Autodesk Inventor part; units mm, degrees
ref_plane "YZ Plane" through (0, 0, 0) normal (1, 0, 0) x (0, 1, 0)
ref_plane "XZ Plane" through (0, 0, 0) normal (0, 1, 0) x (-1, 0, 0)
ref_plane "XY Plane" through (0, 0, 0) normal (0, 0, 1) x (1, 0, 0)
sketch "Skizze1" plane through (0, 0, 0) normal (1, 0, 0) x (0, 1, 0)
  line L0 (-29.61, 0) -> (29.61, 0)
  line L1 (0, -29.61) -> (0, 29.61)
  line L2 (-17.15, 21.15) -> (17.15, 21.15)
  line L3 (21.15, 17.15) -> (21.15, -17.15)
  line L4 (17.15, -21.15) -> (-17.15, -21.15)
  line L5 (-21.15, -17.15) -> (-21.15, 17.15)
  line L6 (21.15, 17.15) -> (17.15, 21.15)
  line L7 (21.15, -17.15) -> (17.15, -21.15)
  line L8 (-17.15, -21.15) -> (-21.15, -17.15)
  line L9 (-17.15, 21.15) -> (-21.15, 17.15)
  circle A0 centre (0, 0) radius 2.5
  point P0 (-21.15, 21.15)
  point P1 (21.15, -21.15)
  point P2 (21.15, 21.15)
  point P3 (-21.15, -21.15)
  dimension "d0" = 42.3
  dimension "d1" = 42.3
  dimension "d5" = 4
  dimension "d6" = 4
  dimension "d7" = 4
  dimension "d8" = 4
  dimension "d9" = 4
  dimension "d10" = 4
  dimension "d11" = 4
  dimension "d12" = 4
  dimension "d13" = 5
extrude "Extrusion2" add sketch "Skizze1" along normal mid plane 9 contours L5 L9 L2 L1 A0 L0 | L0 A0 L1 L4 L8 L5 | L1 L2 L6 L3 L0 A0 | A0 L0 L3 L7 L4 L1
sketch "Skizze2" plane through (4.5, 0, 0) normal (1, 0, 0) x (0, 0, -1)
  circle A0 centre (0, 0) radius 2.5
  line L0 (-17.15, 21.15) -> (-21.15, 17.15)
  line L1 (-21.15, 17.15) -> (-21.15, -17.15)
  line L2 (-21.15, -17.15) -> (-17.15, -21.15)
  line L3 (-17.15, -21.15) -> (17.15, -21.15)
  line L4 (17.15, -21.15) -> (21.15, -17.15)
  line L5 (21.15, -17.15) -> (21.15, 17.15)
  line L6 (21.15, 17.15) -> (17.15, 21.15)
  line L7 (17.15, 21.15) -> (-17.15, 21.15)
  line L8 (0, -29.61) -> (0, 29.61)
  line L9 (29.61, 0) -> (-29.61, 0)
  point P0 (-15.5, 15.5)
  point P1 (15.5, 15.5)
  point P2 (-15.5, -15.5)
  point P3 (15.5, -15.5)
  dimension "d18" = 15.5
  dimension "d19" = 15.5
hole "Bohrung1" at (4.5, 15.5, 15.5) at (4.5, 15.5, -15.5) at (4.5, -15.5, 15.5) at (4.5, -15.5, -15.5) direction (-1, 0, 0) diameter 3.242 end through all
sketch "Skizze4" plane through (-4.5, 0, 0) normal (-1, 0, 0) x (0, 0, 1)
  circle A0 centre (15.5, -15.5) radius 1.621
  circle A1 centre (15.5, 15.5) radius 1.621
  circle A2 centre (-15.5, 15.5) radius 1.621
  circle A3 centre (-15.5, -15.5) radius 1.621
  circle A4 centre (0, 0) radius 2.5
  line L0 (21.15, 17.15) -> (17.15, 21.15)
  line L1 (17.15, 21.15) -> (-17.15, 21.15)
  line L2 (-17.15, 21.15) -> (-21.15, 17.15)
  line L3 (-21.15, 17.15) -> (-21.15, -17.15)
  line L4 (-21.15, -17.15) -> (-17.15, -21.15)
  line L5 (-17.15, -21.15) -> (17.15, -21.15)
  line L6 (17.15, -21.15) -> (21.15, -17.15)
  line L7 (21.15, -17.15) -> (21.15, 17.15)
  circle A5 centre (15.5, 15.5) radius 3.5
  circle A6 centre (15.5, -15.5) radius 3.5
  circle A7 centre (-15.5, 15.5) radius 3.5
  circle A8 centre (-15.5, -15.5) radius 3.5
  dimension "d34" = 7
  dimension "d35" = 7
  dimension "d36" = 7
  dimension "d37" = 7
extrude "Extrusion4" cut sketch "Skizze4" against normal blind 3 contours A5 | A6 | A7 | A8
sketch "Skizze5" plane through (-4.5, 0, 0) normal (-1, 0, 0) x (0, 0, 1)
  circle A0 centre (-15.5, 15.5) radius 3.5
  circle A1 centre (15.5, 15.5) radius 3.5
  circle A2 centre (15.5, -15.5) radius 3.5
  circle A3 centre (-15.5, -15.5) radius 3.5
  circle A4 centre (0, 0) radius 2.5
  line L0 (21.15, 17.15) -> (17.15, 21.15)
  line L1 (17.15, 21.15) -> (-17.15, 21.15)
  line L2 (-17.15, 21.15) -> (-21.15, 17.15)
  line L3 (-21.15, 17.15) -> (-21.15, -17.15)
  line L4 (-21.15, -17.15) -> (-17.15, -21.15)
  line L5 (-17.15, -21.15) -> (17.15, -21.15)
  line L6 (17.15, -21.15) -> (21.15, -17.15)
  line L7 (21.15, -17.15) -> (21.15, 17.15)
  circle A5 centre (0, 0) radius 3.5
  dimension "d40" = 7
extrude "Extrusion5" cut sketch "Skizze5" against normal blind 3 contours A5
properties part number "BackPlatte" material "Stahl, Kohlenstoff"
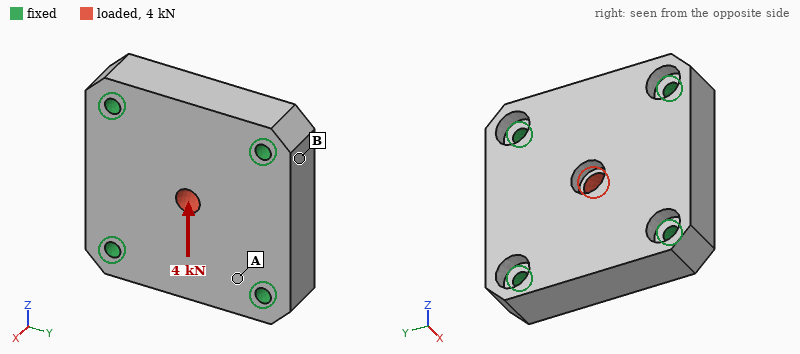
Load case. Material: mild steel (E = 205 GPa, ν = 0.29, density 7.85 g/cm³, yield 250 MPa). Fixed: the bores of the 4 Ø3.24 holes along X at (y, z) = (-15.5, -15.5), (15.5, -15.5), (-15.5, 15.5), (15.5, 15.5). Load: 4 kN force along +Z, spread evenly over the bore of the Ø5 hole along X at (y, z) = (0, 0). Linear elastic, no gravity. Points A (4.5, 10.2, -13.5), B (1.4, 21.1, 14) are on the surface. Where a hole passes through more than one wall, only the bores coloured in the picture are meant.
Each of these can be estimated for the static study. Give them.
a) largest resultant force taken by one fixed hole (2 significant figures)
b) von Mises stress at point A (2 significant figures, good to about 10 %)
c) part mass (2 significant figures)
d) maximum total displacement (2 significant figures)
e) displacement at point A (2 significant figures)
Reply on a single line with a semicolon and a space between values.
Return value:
1.1 kN; 15 MPa; 120 g; 2.4 µm; 0.61 µm
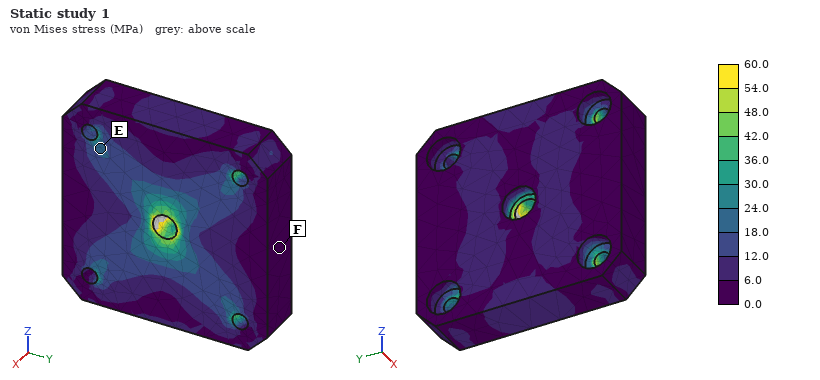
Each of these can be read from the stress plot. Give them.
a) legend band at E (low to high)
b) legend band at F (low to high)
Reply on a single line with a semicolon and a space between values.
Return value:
18.0 to 24.0 MPa; 0.0 to 6.0 MPa
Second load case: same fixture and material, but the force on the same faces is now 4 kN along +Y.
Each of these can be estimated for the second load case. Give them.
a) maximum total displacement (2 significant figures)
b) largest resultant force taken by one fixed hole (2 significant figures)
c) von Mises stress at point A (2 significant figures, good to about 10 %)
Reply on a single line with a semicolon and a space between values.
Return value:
2.4 µm; 1.1 kN; 17 MPa
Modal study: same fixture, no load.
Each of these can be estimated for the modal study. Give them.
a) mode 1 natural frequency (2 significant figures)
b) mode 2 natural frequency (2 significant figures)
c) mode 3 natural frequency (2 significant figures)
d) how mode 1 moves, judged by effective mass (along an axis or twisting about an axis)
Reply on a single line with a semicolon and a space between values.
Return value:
21 kHz; 31 kHz; 31 kHz; along X
